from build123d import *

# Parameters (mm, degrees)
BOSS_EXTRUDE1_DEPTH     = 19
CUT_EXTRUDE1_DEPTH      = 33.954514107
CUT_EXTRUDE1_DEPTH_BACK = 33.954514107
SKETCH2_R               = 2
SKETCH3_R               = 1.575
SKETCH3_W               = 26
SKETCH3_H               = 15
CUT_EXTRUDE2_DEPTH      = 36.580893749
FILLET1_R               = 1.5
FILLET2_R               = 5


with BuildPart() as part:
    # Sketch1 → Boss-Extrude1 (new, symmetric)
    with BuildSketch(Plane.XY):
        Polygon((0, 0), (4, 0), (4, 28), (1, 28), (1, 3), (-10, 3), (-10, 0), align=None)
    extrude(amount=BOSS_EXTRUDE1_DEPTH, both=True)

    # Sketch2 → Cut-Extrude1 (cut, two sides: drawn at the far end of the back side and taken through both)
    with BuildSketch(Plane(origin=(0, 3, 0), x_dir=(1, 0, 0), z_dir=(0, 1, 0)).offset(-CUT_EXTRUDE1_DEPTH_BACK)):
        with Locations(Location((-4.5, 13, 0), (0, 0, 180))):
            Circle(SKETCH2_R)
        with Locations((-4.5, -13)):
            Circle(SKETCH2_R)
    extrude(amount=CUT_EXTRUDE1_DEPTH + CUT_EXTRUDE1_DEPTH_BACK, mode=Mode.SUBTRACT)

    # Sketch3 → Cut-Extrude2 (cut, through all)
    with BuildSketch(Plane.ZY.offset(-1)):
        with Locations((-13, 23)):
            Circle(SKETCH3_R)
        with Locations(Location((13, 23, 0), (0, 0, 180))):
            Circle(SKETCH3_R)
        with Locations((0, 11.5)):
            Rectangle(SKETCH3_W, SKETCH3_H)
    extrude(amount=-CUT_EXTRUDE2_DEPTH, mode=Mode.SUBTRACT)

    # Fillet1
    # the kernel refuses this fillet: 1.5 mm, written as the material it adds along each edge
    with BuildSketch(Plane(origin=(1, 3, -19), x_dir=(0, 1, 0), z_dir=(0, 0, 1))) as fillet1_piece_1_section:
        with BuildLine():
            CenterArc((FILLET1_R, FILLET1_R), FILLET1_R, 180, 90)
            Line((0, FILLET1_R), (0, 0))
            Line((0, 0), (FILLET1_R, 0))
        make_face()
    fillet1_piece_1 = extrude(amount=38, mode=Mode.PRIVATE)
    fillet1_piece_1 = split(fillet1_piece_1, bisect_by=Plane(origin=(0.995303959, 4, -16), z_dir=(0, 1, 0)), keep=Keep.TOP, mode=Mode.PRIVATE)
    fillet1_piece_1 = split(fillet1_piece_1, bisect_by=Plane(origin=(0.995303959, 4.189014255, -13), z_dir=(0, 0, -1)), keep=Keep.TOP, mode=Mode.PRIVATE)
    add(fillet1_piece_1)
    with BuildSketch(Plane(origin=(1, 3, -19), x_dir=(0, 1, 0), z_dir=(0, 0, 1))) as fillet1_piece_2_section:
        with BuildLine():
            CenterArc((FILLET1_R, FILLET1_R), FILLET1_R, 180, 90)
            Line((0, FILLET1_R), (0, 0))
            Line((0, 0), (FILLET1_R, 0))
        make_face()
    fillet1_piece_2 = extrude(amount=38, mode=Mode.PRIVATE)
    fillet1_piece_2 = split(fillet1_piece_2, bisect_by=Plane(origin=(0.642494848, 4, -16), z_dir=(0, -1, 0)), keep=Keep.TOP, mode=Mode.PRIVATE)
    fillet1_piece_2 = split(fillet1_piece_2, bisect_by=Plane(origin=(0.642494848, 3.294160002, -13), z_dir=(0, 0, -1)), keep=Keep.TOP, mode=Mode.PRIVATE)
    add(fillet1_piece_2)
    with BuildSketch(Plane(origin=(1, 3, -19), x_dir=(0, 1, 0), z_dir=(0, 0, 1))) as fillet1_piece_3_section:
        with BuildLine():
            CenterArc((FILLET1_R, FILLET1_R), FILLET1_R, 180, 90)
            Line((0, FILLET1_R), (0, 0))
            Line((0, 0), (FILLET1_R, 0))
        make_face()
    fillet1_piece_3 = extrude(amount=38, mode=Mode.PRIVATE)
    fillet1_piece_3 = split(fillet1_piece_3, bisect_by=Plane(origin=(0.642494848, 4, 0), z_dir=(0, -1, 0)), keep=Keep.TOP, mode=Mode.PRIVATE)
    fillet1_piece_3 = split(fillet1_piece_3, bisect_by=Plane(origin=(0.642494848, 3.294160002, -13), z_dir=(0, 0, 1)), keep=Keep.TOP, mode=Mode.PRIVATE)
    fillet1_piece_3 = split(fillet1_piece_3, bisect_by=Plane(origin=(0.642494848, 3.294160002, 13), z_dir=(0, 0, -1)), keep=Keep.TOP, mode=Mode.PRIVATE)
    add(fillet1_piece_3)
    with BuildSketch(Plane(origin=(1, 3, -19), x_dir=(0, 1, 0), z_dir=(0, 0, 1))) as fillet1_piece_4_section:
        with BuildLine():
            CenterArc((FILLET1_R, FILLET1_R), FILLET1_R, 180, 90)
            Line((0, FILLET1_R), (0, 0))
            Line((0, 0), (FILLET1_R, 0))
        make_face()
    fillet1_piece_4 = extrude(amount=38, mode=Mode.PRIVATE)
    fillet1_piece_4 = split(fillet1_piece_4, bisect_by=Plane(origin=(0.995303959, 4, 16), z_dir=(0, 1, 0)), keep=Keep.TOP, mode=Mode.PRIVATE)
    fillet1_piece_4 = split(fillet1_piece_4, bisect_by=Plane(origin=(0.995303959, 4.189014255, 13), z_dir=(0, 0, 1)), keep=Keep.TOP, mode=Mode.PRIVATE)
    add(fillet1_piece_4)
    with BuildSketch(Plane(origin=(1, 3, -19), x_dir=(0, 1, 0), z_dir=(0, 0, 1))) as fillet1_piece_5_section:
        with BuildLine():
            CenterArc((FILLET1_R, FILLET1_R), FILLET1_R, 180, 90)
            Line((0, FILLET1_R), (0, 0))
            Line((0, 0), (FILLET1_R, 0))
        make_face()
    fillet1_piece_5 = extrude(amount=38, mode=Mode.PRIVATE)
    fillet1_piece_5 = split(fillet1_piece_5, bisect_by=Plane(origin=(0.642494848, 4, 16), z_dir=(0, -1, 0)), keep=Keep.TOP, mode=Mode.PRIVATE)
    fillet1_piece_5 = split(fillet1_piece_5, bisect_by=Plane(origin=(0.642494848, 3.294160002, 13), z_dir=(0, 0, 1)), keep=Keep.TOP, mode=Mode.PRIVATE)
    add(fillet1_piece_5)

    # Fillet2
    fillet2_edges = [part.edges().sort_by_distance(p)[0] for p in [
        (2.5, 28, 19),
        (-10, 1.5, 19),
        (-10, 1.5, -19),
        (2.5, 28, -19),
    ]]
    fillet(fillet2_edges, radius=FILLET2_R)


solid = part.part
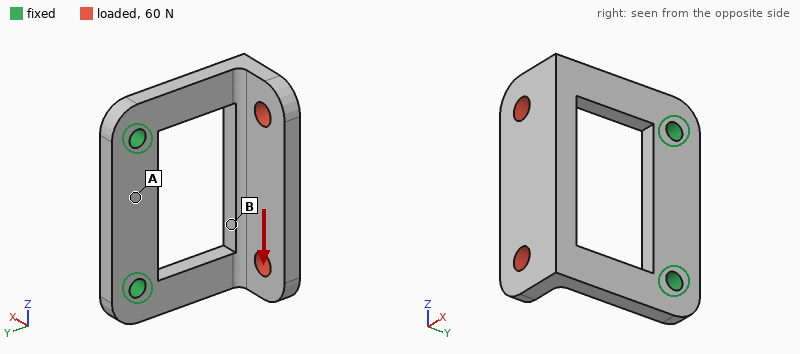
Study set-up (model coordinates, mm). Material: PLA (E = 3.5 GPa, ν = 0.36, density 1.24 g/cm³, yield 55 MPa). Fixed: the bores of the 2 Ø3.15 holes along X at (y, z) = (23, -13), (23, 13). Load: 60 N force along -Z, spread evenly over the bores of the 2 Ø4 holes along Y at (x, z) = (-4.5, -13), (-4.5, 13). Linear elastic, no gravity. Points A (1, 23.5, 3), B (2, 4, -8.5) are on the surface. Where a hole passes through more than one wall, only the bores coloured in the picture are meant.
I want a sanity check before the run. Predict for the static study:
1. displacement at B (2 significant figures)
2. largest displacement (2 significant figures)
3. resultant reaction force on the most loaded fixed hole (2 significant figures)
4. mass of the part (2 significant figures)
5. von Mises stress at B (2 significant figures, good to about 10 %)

0.28 mm
0.52 mm
43 N
3.9 g
9.0 MPa
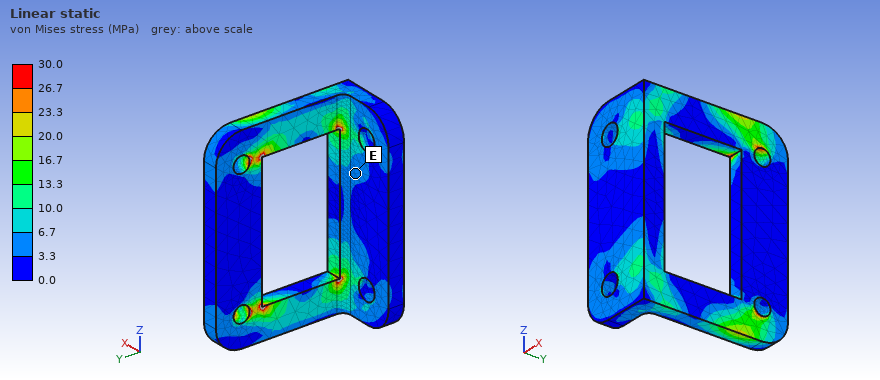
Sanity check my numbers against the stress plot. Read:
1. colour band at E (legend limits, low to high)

3.3 to 6.7 MPa
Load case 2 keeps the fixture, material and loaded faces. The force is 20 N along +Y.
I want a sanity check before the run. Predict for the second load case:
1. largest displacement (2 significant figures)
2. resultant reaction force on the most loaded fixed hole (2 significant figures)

0.53 mm
10 N
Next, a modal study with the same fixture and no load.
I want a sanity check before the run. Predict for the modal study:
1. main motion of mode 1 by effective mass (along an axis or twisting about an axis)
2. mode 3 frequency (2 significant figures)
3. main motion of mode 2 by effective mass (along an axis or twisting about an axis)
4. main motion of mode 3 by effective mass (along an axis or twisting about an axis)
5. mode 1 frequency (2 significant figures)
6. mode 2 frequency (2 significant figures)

along X
1900 Hz
along Z
along Z
560 Hz
1200 Hz
